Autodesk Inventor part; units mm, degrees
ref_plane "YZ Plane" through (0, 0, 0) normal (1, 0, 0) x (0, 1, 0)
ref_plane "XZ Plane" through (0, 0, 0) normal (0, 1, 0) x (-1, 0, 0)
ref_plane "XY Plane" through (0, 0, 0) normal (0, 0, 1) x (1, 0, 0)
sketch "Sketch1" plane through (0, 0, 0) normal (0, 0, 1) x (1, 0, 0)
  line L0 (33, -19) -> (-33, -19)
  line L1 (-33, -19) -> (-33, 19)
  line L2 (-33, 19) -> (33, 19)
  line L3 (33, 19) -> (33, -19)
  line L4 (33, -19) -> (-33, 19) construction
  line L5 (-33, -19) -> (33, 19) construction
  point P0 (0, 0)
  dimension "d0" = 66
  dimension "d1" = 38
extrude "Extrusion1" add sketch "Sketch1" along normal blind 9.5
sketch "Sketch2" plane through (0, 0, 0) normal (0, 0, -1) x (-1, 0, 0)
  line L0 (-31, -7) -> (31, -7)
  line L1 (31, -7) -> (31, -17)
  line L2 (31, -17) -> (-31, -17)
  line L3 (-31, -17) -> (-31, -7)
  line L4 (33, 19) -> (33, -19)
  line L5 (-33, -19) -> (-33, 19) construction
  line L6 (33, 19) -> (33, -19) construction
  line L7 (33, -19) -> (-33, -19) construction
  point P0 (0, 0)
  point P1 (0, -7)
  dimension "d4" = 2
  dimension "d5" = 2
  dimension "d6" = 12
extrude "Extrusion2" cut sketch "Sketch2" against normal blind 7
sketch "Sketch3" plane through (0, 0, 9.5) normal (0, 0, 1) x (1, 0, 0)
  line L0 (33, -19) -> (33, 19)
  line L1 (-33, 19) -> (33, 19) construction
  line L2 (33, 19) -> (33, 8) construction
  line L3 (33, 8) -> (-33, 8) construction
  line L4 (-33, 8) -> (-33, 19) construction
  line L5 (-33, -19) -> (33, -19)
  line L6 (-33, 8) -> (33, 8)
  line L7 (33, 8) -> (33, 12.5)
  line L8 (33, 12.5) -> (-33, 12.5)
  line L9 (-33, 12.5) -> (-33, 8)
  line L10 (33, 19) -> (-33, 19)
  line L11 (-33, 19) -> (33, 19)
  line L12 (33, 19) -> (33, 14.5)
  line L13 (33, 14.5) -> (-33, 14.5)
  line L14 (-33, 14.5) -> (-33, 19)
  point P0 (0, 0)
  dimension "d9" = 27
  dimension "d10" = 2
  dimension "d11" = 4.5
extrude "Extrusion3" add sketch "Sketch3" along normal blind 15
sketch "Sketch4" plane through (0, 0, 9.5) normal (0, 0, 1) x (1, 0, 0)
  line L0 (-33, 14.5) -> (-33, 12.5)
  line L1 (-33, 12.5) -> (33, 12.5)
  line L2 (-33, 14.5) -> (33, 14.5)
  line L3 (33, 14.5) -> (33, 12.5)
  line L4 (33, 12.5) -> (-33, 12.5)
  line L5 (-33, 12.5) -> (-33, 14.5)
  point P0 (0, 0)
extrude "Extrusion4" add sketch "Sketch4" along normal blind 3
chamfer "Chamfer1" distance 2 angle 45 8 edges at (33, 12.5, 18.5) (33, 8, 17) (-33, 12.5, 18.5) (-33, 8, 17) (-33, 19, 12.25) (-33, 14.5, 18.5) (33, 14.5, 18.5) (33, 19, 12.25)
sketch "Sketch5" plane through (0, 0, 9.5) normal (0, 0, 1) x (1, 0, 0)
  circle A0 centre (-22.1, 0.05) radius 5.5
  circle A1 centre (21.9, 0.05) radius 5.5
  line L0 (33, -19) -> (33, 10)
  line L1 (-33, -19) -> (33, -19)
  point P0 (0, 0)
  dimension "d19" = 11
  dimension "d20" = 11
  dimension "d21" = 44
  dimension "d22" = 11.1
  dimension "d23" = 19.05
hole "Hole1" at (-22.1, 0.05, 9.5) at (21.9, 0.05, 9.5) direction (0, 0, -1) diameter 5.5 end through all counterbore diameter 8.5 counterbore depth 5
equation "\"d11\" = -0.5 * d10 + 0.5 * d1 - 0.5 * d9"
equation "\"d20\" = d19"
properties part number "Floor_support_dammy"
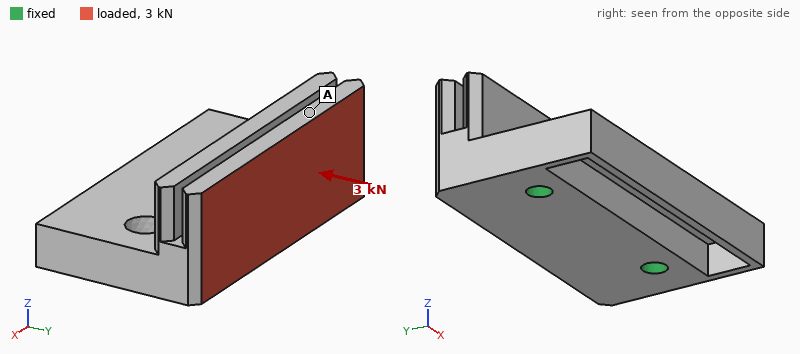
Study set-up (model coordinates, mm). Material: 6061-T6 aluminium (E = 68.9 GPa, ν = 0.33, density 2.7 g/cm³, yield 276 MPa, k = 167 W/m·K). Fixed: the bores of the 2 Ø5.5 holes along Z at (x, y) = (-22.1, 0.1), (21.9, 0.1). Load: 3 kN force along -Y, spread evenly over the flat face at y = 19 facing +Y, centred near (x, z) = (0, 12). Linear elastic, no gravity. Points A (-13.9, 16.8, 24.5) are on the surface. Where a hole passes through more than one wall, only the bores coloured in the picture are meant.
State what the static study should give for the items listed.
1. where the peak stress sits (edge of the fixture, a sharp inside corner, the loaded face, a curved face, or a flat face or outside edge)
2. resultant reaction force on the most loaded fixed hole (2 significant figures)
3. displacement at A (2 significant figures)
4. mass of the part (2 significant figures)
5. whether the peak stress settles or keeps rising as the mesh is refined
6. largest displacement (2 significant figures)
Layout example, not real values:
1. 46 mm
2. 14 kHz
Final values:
1. edge of the fixture
2. 1.5 kN
3. 0.095 mm
4. 75 g
5. keeps rising
6. 0.10 mm
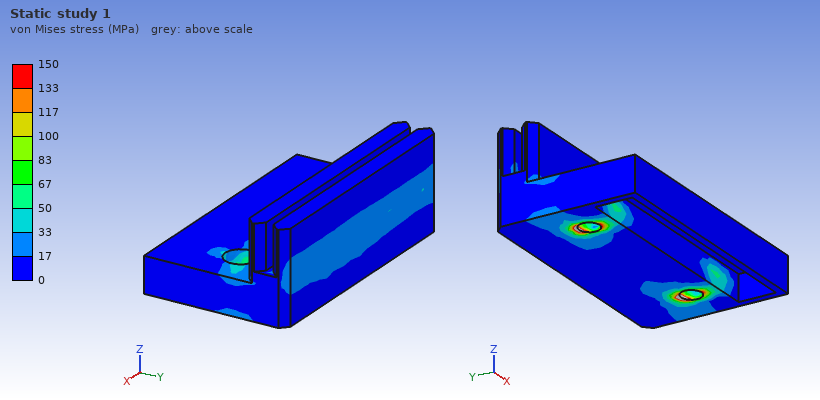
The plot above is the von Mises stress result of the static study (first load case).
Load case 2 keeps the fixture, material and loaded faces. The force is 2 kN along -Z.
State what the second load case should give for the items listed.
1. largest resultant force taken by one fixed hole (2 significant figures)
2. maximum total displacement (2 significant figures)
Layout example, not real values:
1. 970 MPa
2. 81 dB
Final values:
1. 1.0 kN
2. 0.10 mm
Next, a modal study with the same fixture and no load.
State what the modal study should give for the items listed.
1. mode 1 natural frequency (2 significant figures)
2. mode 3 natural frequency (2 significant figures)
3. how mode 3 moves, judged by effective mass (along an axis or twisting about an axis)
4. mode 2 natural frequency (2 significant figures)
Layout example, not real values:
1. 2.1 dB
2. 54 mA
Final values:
1. 4300 Hz
2. 8700 Hz
3. along Z
4. 8300 Hz
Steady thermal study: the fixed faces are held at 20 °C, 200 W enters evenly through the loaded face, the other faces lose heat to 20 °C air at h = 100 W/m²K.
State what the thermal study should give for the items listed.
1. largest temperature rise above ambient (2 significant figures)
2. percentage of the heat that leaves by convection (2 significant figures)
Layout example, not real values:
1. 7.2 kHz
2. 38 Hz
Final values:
1. 62 K
2. 14 %
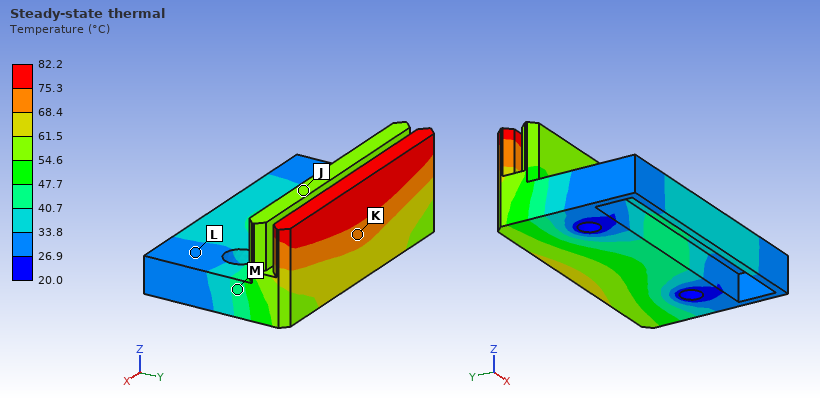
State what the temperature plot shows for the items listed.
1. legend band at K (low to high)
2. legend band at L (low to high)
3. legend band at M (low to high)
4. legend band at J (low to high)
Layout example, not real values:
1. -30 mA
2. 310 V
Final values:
1. 68.4 to 75.3 °C
2. 26.9 to 33.8 °C
3. 40.7 to 47.7 °C
4. 54.6 to 61.5 °C
